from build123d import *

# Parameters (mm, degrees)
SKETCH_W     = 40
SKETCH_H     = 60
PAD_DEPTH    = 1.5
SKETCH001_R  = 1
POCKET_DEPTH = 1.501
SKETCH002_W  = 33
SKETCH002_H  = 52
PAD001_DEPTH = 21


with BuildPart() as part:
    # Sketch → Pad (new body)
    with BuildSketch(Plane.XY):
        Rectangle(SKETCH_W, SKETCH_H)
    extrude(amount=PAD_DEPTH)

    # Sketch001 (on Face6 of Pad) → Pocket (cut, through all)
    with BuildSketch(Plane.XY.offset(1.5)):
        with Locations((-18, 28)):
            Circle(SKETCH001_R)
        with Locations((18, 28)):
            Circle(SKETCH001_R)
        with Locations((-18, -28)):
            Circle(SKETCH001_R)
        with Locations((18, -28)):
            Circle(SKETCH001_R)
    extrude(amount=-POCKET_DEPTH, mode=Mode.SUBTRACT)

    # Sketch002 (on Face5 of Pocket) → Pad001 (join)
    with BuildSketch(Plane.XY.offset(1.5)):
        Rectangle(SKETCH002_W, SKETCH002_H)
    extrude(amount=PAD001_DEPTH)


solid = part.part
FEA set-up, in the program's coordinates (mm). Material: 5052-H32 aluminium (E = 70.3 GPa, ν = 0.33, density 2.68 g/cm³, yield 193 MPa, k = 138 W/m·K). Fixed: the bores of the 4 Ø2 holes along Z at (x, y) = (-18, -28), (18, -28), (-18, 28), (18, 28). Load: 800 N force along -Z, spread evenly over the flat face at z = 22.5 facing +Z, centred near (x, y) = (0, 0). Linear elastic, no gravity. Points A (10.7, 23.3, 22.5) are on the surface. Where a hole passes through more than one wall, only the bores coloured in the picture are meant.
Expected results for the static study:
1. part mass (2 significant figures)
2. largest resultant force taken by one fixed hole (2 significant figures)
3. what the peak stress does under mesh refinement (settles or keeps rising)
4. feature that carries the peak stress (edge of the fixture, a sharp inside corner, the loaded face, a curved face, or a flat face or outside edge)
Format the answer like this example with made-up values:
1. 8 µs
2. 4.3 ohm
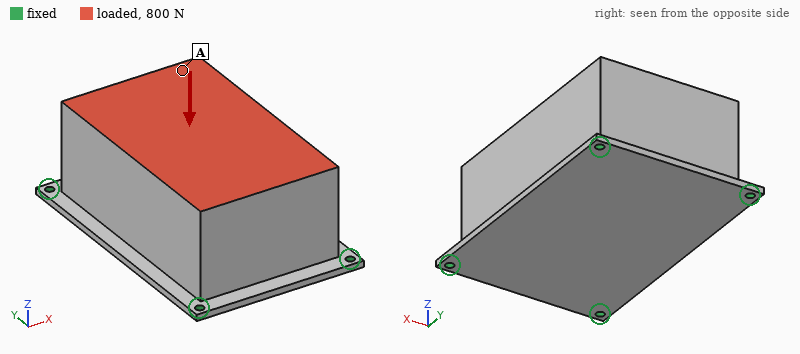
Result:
1. 110 g
2. 230 N
3. keeps rising
4. edge of the fixture
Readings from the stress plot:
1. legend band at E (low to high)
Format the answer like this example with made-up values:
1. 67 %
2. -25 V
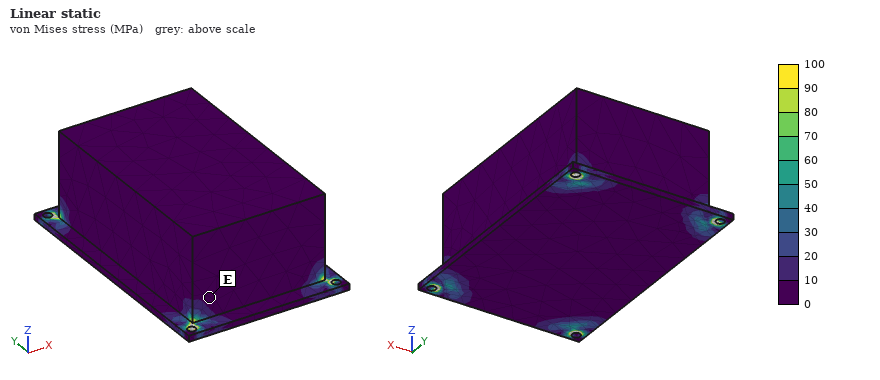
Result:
1. 0 to 10 MPa
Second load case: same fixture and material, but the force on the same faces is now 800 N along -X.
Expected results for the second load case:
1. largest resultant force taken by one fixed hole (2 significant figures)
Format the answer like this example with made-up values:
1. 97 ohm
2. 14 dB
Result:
1. 360 N
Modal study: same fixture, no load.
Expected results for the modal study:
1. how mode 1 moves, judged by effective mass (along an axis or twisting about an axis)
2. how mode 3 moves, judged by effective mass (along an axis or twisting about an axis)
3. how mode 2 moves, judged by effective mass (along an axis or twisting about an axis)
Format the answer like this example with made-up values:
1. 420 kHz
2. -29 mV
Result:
1. along Z
2. along Y
3. along X
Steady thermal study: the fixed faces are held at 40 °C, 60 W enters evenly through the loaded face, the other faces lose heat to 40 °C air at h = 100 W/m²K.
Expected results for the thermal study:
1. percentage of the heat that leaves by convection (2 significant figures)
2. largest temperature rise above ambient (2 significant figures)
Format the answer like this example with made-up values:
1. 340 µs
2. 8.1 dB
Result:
1. 38 %
2. 39 K
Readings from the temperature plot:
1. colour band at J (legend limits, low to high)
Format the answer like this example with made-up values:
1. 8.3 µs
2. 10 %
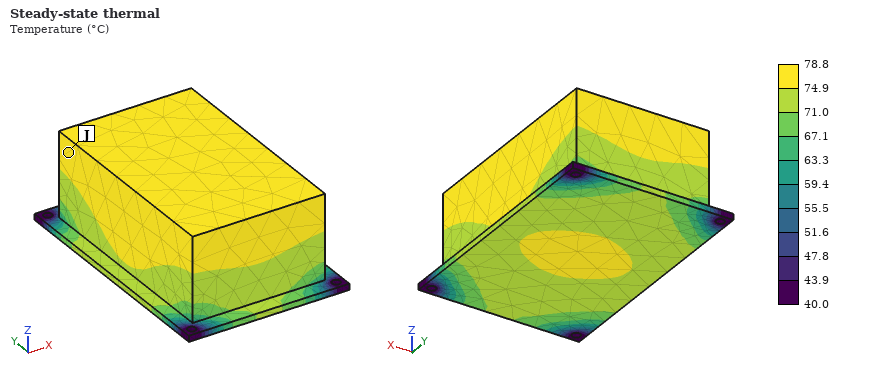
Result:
1. 74.9 to 78.8 °C
